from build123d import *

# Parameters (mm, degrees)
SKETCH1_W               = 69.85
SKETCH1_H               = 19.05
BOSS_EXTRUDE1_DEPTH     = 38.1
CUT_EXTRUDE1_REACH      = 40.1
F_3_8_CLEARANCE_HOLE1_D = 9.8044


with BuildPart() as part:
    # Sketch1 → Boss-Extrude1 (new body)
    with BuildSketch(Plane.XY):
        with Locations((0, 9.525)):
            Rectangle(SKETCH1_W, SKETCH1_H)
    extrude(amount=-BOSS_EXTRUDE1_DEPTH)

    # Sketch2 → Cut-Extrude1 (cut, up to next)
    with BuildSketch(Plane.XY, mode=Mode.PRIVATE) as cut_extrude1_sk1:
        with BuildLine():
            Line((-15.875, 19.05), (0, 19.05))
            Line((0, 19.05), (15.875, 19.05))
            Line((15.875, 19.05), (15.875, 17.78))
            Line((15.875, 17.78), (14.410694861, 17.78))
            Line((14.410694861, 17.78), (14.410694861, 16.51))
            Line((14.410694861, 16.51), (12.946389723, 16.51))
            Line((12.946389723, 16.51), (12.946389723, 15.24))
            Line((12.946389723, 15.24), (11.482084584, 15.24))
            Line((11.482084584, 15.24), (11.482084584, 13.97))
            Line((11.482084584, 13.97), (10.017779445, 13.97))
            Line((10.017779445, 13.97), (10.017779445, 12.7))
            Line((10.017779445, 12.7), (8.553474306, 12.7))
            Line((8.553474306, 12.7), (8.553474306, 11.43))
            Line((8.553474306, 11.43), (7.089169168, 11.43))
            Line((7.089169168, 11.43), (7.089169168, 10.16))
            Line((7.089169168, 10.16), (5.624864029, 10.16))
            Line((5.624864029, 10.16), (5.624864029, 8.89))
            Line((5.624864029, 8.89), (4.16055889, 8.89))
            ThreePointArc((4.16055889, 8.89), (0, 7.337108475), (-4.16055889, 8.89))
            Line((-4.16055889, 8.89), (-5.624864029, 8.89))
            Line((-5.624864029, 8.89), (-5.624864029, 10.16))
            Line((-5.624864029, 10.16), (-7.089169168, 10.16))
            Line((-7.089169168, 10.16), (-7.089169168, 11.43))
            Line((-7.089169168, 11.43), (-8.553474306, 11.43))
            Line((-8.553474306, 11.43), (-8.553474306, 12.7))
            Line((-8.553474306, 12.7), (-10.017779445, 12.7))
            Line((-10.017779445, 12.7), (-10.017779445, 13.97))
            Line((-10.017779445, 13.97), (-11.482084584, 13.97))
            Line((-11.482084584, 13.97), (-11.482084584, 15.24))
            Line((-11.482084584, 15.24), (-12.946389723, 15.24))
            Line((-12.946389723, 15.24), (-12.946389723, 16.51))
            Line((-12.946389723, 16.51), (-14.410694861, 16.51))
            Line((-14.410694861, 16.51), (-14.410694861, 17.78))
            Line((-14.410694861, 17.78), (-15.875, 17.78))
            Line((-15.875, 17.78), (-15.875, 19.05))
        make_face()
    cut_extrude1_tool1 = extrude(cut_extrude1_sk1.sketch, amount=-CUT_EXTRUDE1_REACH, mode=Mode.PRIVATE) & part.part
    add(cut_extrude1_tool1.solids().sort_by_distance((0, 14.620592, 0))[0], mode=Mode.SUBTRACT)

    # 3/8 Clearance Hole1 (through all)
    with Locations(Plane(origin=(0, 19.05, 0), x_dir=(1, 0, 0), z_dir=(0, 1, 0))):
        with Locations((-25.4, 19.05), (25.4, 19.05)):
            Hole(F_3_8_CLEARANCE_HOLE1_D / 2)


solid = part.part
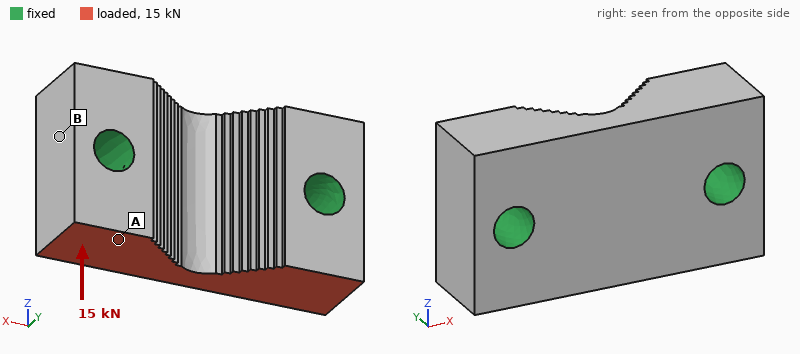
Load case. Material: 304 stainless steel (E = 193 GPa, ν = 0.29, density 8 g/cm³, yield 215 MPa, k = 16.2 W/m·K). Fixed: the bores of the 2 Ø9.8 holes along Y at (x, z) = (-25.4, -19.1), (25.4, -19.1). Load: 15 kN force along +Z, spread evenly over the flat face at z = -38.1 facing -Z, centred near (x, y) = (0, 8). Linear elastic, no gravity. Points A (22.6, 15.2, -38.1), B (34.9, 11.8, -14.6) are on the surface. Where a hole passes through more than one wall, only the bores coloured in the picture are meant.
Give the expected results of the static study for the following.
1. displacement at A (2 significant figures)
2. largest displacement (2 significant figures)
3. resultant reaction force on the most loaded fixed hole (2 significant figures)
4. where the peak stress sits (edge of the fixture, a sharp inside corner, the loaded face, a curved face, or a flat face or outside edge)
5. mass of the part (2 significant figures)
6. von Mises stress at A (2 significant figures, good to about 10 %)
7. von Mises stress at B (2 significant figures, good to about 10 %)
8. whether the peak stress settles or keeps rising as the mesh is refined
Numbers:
1.5 µm
3.4 µm
7.5 kN
edge of the fixture
310 g
16 MPa
5.7 MPa
keeps rising
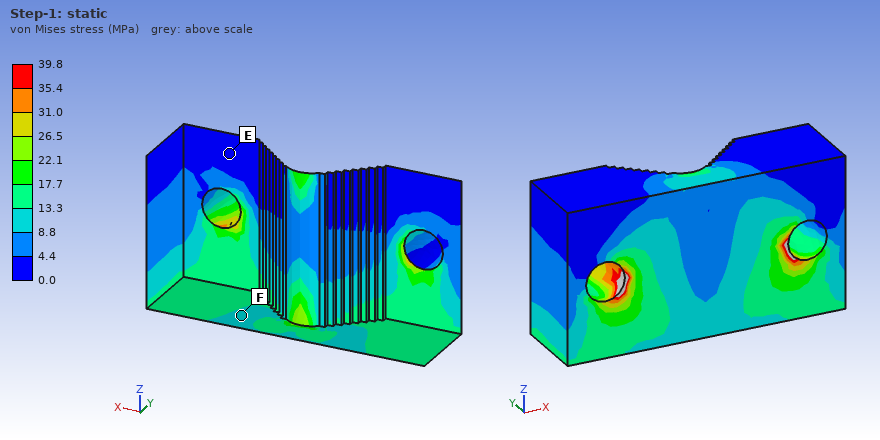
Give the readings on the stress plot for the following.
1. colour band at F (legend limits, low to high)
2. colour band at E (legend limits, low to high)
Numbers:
8.8 to 13.3 MPa
0.0 to 4.4 MPa
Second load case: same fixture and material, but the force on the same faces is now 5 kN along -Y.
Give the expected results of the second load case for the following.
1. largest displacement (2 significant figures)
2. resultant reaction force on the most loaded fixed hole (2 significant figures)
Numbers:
5.0 µm
2.5 kN
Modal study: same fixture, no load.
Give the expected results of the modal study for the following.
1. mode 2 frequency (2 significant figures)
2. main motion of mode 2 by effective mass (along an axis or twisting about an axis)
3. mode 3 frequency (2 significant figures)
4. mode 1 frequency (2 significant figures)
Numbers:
24 kHz
along Y
27 kHz
22 kHz
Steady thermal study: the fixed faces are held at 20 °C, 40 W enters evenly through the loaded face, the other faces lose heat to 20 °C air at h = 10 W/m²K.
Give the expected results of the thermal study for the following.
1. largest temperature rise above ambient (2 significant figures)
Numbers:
47 K
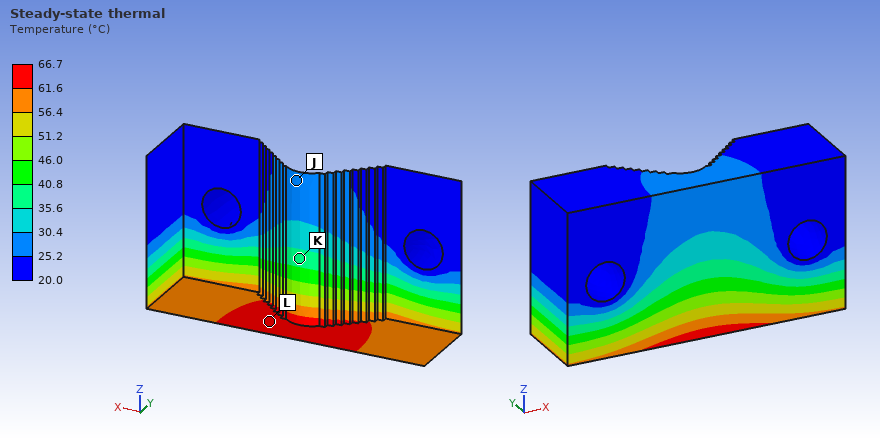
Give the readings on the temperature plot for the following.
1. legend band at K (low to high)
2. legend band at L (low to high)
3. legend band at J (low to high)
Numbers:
35.6 to 40.8 °C
61.6 to 66.7 °C
25.2 to 30.4 °C
